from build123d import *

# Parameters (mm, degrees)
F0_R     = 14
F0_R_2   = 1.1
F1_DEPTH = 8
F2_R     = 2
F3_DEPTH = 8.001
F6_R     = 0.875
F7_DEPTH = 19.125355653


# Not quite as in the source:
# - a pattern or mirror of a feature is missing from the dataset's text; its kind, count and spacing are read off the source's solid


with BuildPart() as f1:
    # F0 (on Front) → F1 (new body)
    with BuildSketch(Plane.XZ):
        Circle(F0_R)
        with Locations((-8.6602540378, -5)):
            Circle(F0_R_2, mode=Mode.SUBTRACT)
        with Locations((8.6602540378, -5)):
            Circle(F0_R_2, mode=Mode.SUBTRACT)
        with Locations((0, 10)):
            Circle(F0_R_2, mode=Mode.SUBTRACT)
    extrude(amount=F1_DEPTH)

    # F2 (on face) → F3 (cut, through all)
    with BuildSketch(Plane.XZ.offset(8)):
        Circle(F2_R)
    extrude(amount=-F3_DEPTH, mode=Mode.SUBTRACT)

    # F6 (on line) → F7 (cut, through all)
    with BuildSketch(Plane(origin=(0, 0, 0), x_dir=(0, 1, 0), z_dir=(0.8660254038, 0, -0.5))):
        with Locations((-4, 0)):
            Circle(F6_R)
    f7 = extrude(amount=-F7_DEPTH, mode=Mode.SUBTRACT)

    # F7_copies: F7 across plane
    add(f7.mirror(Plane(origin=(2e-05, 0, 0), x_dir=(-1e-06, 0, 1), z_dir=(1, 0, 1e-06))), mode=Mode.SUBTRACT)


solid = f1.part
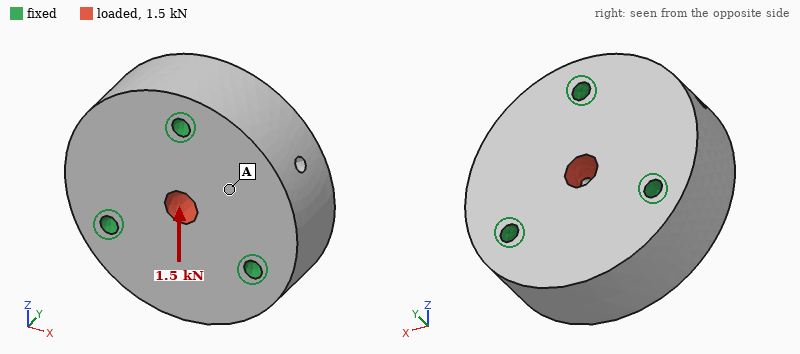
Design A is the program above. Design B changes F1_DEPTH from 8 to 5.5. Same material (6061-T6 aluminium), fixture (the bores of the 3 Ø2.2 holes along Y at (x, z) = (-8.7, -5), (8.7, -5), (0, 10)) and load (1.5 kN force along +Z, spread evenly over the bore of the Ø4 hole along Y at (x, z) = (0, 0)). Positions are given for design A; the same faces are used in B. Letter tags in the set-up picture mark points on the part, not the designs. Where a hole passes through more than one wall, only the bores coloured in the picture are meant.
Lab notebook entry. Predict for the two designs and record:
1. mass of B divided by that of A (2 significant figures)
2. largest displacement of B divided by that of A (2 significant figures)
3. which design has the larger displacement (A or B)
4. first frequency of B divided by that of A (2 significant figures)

0.68
1.5
B
0.83
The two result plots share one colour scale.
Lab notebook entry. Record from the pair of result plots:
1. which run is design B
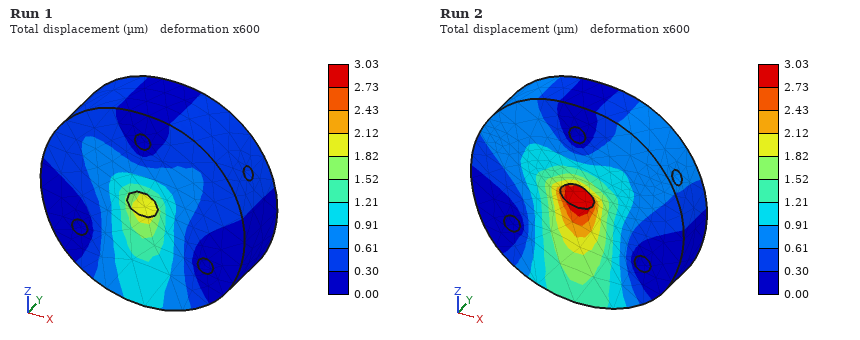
Run 2
